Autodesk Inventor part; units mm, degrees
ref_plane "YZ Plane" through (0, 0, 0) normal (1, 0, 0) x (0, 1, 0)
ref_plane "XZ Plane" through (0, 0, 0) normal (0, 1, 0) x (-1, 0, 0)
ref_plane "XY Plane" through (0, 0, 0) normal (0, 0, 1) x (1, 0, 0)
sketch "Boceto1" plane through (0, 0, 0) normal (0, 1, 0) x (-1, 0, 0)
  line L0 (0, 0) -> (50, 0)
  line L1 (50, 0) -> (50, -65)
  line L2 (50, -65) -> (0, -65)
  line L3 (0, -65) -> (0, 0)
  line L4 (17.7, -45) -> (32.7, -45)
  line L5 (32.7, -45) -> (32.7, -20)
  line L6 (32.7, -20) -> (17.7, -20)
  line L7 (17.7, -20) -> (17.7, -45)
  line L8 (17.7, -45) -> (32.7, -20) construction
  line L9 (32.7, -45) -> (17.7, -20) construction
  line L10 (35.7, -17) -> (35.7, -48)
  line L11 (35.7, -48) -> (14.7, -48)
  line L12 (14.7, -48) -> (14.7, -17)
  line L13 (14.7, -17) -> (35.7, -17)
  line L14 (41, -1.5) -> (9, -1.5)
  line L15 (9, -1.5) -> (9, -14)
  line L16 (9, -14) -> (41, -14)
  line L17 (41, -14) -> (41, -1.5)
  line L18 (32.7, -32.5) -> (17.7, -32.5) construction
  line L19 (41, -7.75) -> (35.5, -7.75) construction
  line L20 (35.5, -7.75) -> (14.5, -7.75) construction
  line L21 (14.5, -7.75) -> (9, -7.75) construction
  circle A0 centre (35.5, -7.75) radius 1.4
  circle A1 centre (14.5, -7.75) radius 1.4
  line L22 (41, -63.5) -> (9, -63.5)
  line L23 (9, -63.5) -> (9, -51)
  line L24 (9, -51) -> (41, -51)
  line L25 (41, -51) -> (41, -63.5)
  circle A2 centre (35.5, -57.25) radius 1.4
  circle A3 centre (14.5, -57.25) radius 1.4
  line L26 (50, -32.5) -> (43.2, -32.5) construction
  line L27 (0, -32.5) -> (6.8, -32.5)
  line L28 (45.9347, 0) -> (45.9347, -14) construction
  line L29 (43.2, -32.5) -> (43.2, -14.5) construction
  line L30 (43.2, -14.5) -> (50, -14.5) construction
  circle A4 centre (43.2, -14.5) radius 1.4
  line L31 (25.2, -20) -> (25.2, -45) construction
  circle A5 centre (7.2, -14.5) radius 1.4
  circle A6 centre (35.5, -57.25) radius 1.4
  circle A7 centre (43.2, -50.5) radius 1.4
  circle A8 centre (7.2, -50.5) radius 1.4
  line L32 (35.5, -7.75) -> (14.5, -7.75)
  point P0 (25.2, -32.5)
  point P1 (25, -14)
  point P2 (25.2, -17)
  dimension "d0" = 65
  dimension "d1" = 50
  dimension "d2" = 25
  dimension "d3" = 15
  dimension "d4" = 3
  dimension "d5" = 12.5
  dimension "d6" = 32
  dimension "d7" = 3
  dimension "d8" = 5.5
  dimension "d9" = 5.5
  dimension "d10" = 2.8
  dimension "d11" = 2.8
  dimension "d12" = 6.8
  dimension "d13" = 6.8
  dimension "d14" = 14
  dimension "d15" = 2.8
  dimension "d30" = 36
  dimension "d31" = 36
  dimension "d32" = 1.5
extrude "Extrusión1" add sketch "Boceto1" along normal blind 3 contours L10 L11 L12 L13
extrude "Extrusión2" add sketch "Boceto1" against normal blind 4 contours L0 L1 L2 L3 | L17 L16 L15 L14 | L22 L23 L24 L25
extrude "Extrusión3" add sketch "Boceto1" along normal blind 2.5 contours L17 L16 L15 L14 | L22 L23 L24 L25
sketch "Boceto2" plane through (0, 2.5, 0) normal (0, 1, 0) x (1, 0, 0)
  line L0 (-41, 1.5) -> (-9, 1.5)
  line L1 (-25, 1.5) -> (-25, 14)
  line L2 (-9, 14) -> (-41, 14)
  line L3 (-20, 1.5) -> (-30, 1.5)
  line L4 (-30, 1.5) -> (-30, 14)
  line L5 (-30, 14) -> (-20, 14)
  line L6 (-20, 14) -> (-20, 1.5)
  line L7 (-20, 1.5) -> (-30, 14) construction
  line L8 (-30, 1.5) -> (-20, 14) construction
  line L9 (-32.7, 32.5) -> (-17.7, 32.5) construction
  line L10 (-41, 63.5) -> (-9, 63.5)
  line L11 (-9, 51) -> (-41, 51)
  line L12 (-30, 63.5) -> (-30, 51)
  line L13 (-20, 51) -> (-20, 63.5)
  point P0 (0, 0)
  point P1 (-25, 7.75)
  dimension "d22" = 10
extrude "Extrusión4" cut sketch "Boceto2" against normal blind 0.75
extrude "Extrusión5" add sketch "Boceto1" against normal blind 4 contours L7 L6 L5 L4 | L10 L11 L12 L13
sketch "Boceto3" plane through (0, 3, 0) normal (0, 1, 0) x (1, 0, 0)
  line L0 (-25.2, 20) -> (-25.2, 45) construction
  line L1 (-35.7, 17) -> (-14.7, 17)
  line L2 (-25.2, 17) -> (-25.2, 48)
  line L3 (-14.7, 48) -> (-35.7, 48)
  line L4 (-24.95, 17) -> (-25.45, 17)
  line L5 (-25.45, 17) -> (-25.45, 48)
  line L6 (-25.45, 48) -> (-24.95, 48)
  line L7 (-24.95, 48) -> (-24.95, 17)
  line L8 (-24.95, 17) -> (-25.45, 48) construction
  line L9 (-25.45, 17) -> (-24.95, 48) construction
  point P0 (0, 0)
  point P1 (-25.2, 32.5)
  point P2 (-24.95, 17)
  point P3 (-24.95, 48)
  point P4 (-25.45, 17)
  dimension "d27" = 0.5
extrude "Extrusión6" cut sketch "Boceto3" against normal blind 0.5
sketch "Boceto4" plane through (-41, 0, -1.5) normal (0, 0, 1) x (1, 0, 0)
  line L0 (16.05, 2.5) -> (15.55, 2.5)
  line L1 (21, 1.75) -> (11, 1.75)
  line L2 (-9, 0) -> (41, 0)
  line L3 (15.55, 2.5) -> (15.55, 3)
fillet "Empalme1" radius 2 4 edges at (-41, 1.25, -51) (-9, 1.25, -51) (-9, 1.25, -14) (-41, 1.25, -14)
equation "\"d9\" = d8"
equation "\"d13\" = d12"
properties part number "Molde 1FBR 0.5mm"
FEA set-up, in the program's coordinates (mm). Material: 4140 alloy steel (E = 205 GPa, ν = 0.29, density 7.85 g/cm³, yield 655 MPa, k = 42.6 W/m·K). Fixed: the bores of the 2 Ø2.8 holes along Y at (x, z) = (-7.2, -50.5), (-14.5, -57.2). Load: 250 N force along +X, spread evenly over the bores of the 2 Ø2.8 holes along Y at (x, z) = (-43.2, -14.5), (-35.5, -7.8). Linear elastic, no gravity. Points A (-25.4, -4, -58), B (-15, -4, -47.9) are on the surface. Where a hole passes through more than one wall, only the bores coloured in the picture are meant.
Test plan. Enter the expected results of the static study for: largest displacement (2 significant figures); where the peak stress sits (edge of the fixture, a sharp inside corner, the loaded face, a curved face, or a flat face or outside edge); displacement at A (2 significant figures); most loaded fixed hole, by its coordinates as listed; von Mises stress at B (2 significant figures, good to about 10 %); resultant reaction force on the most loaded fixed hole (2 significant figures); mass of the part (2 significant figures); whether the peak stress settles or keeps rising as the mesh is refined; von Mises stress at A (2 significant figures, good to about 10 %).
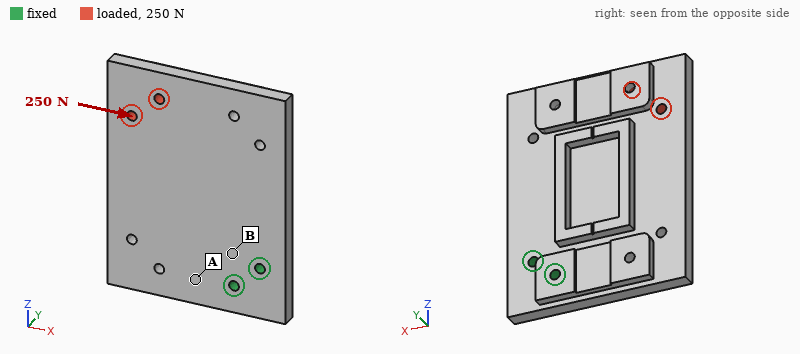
12 µm
edge of the fixture
2.0 µm
(-7.2, -50.5)
13 MPa
940 N
120 g
keeps rising
6.0 MPa
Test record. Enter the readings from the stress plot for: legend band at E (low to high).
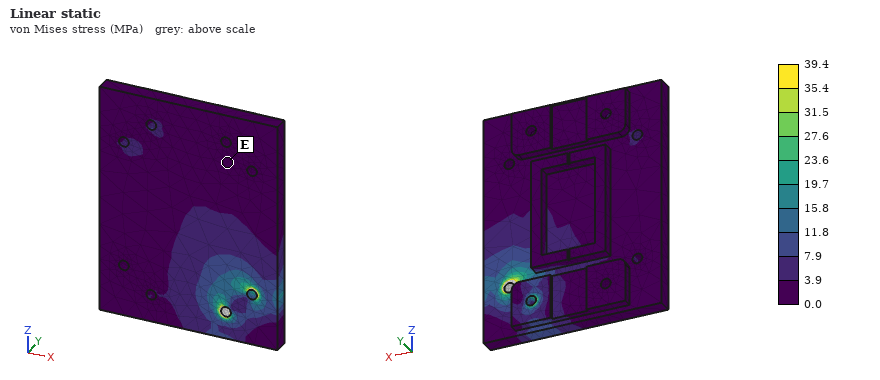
0.0 to 3.9 MPa
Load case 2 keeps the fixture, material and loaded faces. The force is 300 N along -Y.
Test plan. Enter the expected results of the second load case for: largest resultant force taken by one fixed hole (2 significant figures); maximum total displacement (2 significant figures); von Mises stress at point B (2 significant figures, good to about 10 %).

180 N
0.28 mm
110 MPa
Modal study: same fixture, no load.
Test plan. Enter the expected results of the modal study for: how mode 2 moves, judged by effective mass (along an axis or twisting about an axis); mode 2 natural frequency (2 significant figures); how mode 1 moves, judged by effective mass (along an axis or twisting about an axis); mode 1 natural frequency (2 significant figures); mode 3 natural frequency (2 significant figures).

twisting about Z
2400 Hz
along Y
1000 Hz
3400 Hz
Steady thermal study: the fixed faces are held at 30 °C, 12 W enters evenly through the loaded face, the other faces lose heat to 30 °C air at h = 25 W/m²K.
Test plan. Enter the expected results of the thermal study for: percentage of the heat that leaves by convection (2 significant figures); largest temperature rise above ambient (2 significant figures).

45 %
63 K
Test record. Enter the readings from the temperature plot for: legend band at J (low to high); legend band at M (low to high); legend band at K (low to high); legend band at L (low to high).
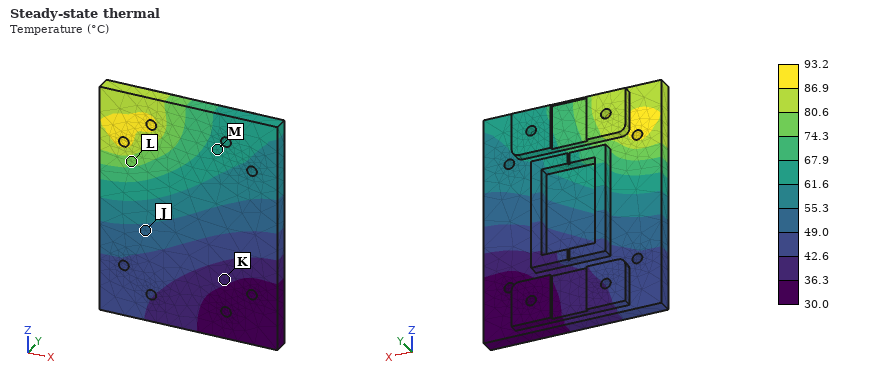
49.0 to 55.3 °C
61.6 to 67.9 °C
36.3 to 42.6 °C
74.3 to 80.6 °C
